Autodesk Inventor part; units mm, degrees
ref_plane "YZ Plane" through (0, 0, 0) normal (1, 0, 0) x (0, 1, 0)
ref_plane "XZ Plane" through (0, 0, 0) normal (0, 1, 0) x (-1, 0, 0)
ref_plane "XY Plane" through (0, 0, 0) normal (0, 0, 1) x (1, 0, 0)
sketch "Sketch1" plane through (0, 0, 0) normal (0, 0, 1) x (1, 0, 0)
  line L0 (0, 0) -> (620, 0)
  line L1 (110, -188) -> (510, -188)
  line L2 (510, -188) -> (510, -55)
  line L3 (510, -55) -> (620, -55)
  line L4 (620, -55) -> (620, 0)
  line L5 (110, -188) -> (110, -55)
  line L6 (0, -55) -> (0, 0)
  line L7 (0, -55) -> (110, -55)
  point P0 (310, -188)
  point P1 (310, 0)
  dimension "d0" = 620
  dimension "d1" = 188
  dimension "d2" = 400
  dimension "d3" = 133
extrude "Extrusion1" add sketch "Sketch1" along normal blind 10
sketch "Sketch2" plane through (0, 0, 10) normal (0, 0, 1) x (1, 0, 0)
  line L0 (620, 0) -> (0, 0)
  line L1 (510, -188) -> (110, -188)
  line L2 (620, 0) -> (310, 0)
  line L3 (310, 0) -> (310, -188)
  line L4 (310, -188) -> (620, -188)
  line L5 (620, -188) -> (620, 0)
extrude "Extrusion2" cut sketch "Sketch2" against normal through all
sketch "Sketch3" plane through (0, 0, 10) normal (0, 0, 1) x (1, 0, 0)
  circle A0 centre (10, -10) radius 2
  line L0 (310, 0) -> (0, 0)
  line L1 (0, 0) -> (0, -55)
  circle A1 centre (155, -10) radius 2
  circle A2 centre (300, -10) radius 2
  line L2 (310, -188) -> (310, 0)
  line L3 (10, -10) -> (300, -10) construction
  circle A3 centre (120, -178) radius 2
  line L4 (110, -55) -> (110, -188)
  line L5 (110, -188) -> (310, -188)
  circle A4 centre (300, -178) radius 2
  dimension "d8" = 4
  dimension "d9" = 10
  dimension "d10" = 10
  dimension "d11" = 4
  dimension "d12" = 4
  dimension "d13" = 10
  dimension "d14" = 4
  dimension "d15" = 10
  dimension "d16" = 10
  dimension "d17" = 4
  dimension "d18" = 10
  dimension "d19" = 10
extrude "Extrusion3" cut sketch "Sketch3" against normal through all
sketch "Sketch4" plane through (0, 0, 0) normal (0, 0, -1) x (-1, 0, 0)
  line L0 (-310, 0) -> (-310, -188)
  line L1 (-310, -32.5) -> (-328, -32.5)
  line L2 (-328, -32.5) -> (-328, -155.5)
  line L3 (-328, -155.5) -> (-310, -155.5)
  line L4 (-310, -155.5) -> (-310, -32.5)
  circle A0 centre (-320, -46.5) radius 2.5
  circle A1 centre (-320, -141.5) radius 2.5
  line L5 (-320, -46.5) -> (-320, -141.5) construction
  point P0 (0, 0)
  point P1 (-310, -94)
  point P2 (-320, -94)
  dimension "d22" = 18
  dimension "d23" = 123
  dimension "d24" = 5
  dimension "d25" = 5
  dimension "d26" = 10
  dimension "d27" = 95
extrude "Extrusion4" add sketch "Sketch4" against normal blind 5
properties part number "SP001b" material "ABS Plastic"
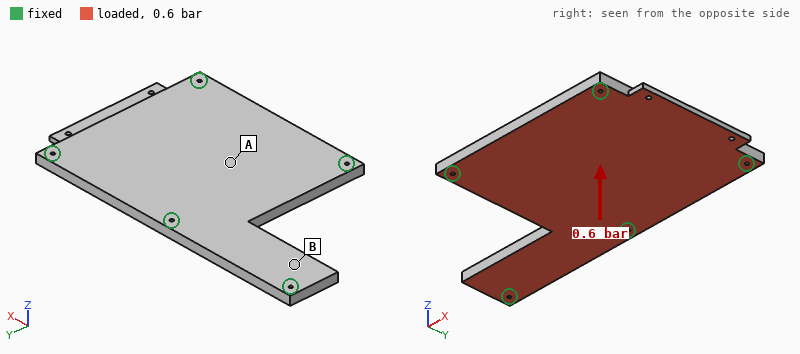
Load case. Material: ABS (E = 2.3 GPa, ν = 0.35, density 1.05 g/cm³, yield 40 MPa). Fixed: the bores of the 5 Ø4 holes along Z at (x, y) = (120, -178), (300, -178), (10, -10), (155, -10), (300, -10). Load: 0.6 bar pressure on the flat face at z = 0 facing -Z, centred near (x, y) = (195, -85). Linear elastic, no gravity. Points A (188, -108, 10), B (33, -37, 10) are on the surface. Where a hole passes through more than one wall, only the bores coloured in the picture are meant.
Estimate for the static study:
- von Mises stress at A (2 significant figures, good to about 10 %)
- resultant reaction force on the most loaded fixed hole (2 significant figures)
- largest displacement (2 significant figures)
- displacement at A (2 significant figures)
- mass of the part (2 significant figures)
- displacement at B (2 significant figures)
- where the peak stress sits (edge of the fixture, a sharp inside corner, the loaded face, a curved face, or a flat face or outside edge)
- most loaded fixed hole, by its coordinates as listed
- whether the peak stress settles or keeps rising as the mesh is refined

6.1 MPa
810 N
2.2 mm
2.1 mm
470 g
0.57 mm
edge of the fixture
(155, -10)
keeps rising
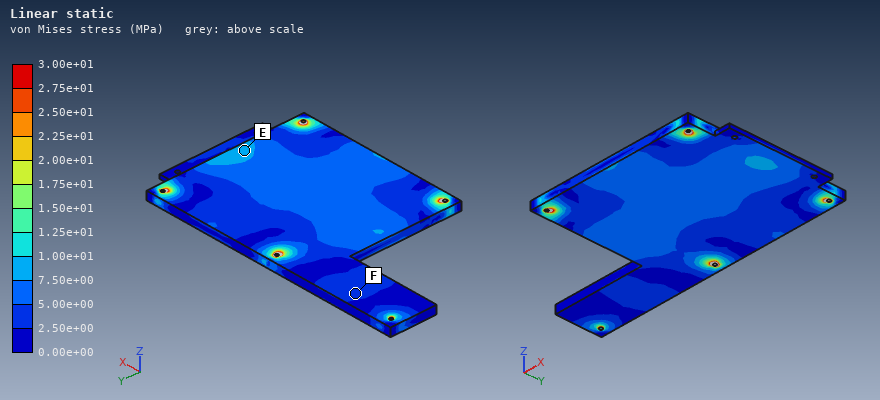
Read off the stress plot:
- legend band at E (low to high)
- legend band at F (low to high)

7.50e+00 to 1.00e+01 MPa
2.50e+00 to 5.00e+00 MPa
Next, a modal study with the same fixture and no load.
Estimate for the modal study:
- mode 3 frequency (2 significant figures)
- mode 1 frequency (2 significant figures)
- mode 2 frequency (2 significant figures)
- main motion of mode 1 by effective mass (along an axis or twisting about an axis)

480 Hz
310 Hz
450 Hz
along Z
